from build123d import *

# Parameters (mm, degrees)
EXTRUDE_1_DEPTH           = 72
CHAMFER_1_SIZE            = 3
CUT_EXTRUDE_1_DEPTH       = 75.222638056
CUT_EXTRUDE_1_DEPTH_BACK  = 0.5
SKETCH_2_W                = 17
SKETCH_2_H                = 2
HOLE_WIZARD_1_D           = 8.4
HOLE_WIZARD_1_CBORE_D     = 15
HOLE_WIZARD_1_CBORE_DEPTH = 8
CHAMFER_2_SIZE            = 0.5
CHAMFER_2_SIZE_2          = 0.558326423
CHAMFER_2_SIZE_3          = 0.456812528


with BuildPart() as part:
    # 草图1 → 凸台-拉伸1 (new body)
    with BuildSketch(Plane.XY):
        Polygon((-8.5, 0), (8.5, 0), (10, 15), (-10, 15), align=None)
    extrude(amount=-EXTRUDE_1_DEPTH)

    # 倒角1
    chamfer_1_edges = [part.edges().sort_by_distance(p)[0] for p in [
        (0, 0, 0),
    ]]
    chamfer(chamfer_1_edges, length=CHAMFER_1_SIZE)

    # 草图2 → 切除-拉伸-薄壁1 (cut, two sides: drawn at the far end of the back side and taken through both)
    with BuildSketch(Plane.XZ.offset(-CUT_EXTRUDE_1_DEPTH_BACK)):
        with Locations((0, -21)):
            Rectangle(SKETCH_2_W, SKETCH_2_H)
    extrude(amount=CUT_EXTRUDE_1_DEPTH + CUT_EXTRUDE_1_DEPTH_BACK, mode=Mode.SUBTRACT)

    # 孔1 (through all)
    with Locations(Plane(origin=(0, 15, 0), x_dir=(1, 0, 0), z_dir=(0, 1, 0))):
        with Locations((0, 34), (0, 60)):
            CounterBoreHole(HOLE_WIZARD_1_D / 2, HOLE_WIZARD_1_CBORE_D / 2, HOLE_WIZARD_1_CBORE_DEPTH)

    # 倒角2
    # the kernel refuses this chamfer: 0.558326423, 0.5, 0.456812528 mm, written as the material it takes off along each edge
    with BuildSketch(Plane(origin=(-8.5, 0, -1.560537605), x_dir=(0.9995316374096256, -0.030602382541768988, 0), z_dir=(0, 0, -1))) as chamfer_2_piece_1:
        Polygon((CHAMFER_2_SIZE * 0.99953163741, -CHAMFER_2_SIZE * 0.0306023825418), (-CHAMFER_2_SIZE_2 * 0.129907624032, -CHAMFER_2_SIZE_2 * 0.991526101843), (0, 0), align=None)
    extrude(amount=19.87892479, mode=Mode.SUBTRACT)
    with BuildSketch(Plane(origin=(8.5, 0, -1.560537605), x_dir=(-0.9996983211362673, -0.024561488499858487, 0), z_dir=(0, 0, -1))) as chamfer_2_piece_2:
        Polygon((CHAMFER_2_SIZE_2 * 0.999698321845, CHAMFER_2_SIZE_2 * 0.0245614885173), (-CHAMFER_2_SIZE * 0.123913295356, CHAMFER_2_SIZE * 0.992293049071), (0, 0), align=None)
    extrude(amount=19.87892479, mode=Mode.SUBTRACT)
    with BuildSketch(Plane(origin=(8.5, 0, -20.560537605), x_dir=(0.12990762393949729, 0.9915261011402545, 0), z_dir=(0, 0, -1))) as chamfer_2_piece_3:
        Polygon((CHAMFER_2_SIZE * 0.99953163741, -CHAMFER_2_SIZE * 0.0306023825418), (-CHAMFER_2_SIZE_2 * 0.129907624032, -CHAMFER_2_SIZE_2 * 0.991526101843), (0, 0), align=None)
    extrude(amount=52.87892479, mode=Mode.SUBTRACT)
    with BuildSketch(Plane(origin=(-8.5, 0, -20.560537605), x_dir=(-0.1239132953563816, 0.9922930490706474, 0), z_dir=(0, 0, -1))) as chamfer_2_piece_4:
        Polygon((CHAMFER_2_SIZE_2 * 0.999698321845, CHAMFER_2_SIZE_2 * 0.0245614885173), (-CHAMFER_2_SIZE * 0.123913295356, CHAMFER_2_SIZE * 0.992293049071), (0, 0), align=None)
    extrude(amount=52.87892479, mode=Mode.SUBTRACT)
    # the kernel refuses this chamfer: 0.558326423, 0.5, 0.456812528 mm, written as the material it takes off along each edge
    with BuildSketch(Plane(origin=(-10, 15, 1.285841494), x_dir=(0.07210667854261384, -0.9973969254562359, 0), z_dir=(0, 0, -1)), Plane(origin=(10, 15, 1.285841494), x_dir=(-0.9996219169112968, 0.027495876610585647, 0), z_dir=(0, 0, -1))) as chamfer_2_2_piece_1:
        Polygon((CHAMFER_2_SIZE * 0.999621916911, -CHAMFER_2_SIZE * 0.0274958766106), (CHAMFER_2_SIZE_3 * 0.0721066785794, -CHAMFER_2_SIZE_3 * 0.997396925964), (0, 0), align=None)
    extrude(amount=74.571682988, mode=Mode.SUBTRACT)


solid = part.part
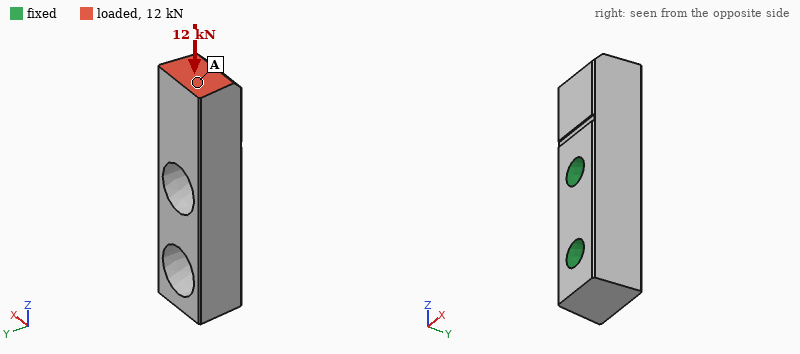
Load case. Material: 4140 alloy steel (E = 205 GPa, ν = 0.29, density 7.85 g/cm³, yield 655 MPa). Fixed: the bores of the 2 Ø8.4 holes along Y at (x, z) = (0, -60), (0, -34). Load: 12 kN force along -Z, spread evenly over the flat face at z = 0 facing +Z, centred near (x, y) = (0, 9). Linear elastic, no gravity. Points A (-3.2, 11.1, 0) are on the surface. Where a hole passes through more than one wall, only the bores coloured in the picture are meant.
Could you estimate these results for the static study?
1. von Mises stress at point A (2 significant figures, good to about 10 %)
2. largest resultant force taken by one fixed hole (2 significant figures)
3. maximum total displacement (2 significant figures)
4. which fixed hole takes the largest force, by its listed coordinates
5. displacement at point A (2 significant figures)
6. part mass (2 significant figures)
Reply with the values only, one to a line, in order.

51 MPa
9.6 kN
51 µm
(0, -34)
47 µm
130 g
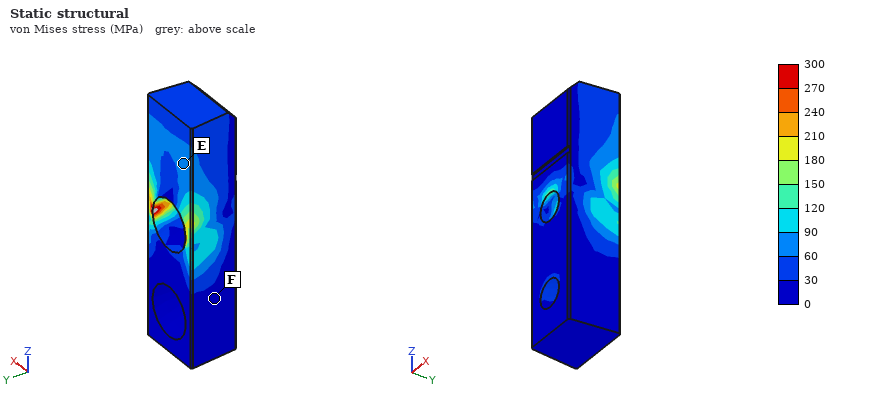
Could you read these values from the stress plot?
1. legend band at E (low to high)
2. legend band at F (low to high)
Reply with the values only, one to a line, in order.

60 to 90 MPa
0 to 30 MPa
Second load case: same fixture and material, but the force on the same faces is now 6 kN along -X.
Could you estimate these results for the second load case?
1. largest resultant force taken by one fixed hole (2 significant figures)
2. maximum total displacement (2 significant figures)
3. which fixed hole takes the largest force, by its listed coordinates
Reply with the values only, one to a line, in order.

8.9 kN
0.10 mm
(0, -34)
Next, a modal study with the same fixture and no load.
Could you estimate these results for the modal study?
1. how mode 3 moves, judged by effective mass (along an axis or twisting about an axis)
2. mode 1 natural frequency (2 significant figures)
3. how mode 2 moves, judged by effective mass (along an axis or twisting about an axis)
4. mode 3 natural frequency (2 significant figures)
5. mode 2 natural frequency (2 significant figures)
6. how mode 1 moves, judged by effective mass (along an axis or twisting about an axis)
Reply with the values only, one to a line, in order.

twisting about Z
6700 Hz
along X
16 kHz
8600 Hz
along Y
